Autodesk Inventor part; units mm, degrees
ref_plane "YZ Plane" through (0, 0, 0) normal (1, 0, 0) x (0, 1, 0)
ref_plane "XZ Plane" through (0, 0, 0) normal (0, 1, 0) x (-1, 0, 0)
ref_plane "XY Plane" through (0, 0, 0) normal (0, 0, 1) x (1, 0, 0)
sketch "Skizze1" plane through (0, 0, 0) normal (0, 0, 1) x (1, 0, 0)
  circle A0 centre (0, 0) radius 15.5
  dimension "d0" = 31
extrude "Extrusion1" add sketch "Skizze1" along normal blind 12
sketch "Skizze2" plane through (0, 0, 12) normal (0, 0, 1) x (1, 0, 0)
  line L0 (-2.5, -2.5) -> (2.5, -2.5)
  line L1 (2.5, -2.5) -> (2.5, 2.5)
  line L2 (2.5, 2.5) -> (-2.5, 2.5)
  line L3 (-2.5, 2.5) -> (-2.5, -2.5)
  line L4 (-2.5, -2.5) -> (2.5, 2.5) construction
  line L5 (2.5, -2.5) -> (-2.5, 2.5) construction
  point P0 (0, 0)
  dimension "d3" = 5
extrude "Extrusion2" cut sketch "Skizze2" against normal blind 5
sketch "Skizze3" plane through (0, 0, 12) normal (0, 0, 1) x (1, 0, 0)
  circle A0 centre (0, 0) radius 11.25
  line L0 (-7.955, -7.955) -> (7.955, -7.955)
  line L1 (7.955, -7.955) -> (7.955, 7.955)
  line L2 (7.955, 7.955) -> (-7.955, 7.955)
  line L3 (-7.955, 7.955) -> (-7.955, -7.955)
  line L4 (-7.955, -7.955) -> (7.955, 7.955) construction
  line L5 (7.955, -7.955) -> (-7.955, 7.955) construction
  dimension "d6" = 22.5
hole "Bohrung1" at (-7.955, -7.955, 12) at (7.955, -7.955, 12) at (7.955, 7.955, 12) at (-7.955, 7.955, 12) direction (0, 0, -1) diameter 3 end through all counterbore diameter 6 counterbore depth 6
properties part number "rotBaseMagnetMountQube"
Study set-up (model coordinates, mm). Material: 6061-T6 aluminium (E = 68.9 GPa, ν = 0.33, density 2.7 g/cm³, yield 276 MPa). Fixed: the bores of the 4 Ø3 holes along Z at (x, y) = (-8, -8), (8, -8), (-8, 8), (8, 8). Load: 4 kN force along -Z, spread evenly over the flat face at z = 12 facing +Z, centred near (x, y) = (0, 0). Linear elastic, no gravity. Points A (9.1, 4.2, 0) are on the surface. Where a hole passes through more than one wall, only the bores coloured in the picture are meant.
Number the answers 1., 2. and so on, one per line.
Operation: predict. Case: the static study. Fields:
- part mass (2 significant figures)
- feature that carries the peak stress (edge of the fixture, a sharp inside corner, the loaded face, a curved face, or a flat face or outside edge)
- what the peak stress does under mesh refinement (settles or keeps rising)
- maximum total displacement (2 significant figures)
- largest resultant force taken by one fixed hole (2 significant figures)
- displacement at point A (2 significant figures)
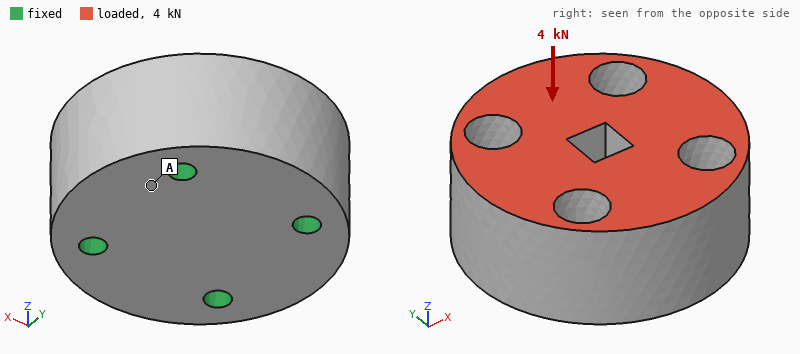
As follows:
1. 22 g
2. edge of the fixture
3. keeps rising
4. 2.8 µm
5. 1.0 kN
6. 1.3 µm
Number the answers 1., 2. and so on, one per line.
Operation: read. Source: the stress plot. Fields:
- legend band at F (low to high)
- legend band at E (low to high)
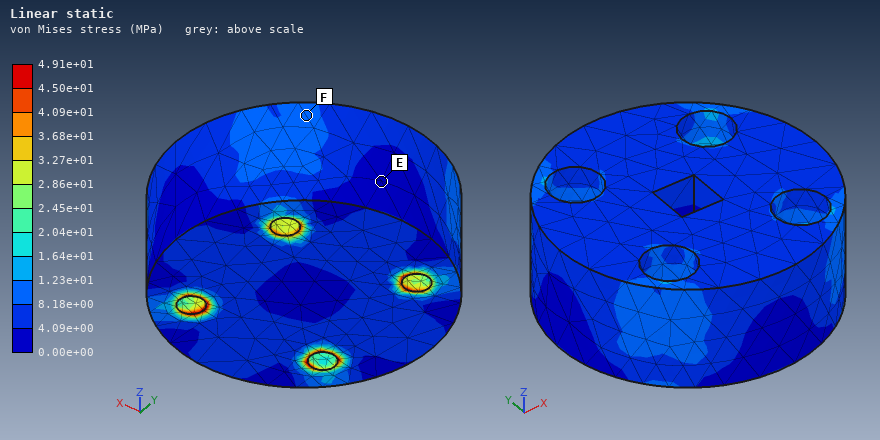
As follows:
1. 8.18e+00 to 1.23e+01 MPa
2. 0.00e+00 to 4.09e+00 MPa
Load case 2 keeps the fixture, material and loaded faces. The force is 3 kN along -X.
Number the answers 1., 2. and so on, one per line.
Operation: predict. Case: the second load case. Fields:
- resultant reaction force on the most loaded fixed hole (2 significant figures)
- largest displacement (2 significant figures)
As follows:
1. 1.0 kN
2. 6.8 µm
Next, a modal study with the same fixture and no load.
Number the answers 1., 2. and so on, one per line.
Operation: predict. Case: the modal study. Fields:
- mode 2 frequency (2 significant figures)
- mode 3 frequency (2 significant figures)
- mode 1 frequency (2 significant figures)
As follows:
1. 45 kHz
2. 51 kHz
3. 45 kHz
